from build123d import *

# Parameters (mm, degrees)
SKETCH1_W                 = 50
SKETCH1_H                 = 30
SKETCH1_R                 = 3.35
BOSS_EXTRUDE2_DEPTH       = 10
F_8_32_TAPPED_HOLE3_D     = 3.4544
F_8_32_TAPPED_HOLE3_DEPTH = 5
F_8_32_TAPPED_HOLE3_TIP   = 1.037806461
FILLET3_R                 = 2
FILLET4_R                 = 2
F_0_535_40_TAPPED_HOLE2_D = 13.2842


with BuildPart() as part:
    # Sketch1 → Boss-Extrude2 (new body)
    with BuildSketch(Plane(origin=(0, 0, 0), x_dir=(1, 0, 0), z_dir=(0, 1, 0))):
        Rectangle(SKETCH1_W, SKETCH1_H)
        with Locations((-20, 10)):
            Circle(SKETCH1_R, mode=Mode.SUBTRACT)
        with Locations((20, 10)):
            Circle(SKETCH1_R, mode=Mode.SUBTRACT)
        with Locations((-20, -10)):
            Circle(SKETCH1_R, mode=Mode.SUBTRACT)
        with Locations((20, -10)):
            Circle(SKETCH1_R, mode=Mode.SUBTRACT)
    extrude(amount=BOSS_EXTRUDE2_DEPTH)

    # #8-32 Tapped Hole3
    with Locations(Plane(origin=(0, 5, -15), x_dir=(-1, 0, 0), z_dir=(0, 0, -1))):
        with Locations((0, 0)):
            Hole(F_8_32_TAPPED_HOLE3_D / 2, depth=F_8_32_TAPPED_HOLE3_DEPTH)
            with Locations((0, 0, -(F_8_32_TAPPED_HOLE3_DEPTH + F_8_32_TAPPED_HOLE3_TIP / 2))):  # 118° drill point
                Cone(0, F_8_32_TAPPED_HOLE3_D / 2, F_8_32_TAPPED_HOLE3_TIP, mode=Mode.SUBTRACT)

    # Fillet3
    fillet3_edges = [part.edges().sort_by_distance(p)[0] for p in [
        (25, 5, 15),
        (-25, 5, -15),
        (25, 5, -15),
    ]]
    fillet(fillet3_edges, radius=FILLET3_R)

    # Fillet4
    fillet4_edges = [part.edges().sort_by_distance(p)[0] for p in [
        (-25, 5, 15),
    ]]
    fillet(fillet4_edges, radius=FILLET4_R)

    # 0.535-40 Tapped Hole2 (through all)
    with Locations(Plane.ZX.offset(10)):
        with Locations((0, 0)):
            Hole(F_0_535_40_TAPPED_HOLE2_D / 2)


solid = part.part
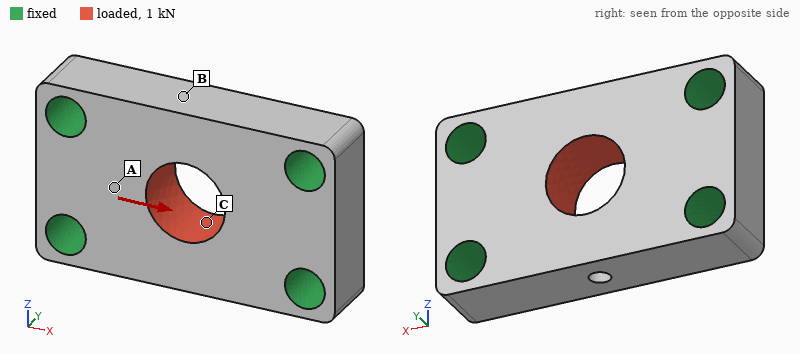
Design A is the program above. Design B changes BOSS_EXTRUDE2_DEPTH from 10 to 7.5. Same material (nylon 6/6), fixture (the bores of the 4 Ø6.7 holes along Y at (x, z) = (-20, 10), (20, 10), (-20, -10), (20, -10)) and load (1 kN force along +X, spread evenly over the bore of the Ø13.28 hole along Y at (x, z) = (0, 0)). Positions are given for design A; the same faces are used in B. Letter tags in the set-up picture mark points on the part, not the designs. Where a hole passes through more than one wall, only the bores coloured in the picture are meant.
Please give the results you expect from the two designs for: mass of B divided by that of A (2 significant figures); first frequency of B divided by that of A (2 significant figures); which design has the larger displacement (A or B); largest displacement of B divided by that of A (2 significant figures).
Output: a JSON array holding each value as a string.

["0.75", "0.86", "B", "1.3"]
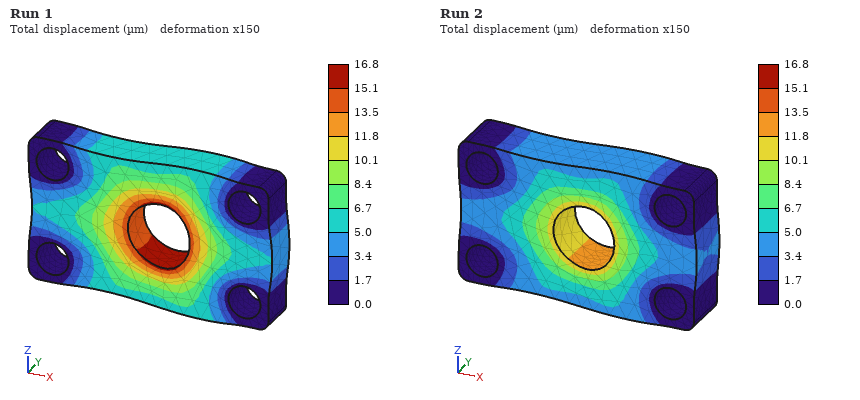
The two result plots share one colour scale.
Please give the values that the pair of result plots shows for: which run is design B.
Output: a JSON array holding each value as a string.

["Run 1"]
